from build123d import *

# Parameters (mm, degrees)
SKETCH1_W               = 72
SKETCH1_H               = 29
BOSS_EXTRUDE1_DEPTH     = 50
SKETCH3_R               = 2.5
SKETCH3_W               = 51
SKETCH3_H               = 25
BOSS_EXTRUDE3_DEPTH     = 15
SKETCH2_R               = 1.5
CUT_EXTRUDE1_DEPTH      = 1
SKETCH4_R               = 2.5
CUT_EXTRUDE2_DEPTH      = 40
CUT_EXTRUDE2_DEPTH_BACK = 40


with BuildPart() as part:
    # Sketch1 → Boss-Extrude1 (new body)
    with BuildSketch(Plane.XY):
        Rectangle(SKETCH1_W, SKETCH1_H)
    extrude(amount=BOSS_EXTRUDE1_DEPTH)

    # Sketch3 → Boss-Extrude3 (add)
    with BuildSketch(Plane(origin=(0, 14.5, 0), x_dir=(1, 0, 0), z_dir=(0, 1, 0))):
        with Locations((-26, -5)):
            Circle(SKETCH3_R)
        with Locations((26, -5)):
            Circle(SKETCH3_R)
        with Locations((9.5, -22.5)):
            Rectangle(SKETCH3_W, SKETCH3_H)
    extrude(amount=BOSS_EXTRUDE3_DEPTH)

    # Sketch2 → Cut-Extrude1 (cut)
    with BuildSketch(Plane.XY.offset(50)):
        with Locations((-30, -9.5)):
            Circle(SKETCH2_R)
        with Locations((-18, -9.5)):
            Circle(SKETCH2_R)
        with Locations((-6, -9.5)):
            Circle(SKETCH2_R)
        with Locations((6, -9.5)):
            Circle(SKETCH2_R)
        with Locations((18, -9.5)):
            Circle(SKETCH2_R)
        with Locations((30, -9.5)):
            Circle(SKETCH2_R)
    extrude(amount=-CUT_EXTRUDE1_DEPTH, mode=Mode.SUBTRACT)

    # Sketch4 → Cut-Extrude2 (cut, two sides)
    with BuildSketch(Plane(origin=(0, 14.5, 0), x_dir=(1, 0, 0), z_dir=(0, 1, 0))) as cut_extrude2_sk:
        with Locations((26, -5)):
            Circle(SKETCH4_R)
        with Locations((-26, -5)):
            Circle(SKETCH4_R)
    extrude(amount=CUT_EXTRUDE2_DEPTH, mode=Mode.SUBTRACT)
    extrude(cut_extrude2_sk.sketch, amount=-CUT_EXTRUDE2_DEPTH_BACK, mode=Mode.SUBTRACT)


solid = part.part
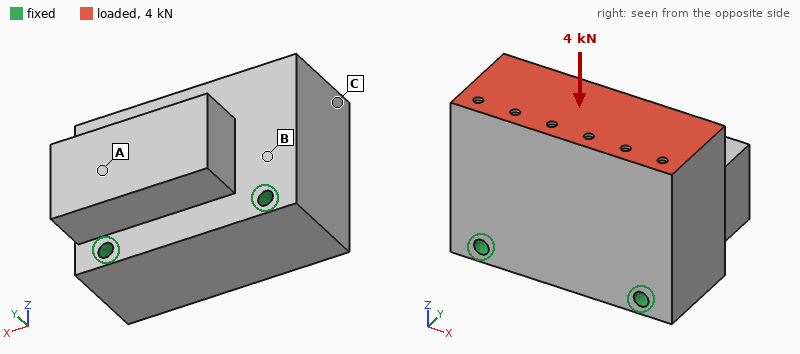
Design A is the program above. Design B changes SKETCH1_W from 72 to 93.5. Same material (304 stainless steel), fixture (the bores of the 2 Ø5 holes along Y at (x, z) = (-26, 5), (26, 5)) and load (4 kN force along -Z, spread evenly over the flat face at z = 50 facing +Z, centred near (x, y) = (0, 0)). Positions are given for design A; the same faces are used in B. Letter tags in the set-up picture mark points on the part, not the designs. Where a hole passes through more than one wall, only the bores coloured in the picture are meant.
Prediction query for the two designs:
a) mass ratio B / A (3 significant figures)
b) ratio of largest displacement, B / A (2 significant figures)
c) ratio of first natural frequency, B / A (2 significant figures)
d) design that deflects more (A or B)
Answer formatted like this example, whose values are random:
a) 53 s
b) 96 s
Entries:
a) 1.25
b) 0.87
c) 0.94
d) A
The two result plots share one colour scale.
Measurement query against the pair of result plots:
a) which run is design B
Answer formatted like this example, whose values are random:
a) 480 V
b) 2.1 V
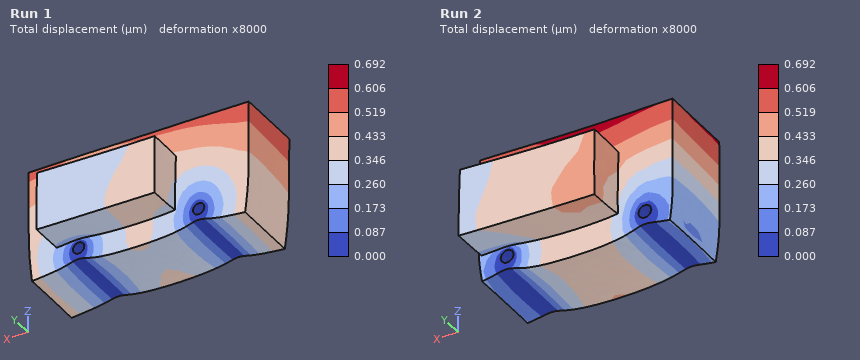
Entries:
a) Run 1
